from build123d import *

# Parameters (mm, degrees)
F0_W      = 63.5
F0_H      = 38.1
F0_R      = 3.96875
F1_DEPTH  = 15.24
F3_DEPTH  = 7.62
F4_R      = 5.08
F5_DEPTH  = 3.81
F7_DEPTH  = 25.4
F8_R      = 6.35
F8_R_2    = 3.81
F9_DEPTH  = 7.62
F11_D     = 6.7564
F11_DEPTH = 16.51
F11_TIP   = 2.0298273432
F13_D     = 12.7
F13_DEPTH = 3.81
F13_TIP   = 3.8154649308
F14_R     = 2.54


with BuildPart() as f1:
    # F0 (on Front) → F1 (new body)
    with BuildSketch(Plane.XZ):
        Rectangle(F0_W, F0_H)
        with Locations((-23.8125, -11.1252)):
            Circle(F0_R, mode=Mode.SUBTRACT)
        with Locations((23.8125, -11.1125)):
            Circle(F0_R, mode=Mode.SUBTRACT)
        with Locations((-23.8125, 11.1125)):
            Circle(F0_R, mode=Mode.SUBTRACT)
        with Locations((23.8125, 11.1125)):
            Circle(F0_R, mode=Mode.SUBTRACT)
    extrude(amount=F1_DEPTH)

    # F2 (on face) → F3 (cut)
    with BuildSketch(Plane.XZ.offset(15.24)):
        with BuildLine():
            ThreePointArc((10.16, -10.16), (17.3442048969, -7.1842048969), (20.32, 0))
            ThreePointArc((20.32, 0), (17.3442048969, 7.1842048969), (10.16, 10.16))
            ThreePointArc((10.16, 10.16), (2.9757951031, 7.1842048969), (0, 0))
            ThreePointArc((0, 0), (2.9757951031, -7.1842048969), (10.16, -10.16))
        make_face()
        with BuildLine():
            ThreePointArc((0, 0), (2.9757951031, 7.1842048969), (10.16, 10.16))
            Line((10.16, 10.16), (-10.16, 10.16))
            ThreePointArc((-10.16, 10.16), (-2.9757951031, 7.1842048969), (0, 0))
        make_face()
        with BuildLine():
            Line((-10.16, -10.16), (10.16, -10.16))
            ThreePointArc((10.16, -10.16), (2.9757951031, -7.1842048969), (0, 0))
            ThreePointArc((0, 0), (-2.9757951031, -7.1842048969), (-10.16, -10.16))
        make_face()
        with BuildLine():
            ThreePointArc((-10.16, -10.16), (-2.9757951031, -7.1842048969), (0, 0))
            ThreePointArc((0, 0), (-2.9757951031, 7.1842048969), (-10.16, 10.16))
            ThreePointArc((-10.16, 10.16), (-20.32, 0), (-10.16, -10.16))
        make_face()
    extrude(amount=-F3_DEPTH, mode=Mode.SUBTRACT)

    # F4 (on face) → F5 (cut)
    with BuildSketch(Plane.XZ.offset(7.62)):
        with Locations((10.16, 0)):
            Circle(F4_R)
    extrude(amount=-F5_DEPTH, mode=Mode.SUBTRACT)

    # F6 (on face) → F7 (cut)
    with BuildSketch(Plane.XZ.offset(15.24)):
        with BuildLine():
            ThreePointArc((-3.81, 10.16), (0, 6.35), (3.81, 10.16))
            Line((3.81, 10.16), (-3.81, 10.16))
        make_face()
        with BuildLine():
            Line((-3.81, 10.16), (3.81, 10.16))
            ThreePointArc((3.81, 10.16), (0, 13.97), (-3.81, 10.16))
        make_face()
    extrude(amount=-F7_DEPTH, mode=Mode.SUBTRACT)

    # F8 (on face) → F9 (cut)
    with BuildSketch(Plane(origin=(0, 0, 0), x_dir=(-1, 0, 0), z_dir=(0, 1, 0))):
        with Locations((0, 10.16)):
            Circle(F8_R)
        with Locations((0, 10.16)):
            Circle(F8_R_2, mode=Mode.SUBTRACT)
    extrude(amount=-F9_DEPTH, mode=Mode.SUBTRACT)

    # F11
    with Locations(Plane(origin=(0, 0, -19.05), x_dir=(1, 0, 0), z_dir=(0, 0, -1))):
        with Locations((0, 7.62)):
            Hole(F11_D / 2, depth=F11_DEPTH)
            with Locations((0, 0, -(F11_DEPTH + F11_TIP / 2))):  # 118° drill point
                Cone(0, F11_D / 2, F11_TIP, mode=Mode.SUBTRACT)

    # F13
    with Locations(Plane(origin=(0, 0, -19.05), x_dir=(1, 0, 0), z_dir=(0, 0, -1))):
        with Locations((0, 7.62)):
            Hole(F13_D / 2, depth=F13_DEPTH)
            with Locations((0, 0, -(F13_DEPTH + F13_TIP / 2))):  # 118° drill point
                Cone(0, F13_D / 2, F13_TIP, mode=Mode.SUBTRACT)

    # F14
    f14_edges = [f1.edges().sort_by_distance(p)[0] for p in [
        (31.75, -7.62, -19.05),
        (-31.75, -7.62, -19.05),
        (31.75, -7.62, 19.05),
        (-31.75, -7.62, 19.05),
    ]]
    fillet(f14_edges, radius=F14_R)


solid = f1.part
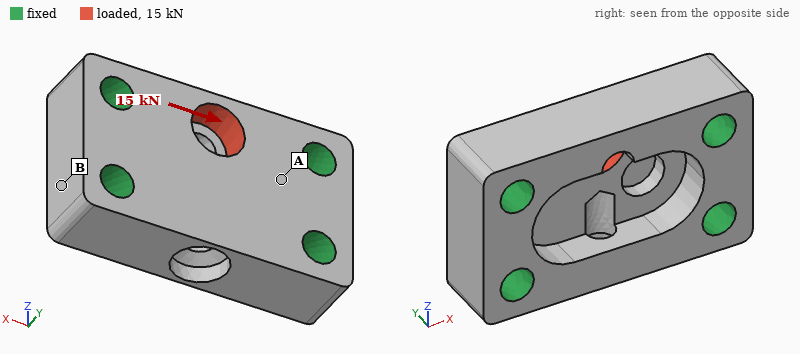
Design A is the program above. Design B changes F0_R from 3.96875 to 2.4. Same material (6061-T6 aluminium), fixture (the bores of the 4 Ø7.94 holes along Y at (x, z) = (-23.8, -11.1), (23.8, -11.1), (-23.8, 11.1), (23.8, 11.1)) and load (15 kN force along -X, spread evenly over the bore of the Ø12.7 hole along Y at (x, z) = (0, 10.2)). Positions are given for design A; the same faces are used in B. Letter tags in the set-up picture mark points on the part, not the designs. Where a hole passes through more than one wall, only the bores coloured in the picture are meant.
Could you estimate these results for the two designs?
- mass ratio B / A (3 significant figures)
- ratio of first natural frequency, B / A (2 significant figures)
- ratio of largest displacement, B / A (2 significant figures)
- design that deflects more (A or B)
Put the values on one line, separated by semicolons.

1.07; 0.89; 1.1; B
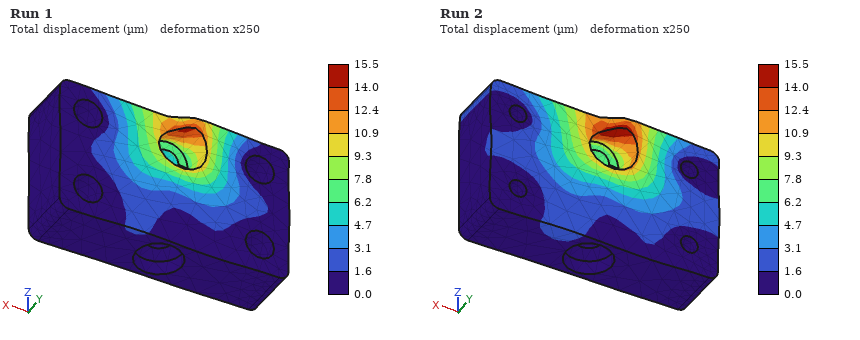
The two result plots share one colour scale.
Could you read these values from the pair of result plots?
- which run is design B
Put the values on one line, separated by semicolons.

Run 2
